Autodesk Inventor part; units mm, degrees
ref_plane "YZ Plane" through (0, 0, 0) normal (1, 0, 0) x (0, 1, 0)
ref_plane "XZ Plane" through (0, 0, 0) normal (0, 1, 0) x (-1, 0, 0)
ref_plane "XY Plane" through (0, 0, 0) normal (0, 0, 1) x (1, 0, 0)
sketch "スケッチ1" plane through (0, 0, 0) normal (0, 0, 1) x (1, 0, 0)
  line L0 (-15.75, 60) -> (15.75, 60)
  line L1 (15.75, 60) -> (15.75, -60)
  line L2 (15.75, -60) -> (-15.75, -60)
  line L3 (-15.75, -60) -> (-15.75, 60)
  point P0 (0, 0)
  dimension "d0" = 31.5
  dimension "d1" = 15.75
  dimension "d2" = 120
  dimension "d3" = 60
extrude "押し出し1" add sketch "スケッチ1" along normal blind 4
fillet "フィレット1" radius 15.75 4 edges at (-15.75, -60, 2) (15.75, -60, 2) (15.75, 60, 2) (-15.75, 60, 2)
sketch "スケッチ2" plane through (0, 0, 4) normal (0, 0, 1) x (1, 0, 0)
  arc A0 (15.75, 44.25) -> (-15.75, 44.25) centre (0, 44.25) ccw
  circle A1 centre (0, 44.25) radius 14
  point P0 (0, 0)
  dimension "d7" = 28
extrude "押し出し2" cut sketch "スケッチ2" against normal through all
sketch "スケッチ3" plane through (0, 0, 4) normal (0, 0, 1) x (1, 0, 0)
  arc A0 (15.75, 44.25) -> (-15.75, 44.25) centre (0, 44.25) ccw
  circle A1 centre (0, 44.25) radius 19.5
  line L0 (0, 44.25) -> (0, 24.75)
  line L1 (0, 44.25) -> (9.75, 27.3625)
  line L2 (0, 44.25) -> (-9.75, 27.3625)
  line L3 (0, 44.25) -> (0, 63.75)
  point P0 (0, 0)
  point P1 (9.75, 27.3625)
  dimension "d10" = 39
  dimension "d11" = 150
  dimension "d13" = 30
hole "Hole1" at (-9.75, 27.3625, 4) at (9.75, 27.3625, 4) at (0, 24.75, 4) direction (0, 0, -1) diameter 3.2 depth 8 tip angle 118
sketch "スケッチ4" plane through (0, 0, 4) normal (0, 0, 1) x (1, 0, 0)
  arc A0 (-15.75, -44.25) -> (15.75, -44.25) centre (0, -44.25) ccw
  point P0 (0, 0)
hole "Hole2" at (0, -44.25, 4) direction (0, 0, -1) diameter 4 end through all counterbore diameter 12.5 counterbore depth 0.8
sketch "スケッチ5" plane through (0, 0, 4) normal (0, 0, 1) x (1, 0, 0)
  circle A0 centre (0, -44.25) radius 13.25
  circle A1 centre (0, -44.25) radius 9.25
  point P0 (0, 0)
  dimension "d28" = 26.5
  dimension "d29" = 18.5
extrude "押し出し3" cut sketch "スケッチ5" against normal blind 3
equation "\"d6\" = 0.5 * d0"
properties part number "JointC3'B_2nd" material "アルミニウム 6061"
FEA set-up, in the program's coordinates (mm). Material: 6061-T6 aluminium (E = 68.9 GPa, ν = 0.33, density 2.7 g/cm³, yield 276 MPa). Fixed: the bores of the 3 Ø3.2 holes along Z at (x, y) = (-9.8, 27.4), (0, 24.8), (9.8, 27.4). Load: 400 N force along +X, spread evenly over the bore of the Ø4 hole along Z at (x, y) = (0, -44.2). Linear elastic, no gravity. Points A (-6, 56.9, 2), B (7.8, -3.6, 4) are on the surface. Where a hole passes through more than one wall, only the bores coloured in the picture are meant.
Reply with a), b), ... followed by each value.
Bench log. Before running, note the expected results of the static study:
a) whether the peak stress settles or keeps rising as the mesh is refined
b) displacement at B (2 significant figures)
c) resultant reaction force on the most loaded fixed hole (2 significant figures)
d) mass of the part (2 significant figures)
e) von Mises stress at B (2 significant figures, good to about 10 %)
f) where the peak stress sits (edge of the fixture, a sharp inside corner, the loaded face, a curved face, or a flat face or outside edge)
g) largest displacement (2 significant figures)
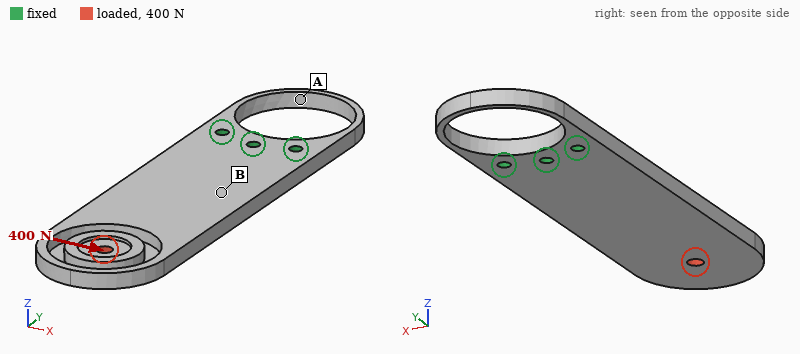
a) keeps rising
b) 0.024 mm
c) 1.3 kN
d) 29 g
e) 13 MPa
f) edge of the fixture
g) 0.12 mm
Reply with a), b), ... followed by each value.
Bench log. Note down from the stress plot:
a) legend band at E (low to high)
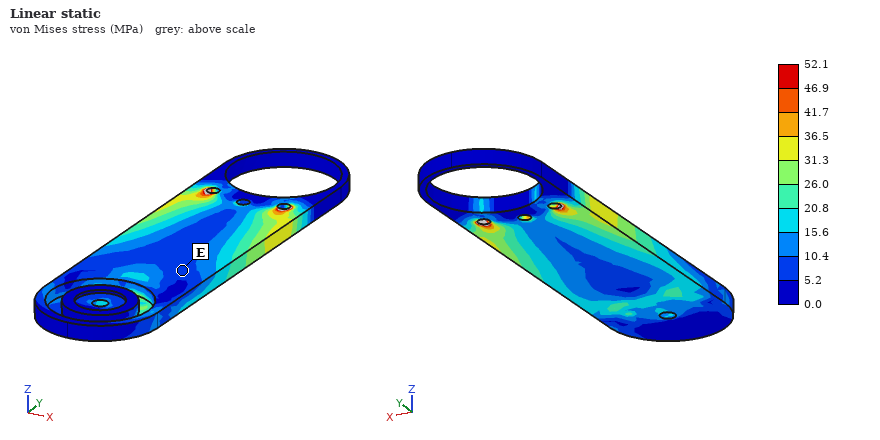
a) 5.2 to 10.4 MPa
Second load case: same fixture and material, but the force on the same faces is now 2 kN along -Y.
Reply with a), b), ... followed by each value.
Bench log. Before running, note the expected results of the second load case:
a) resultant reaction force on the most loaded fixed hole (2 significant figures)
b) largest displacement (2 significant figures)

a) 680 N
b) 0.14 mm
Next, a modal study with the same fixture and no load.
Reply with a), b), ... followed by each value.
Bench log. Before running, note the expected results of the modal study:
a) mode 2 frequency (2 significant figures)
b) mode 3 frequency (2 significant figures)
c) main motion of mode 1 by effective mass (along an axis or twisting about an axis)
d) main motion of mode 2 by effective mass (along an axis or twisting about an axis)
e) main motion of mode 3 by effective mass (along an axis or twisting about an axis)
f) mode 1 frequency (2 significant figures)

a) 2700 Hz
b) 2900 Hz
c) along Z
d) twisting about Y
e) along Z
f) 560 Hz
